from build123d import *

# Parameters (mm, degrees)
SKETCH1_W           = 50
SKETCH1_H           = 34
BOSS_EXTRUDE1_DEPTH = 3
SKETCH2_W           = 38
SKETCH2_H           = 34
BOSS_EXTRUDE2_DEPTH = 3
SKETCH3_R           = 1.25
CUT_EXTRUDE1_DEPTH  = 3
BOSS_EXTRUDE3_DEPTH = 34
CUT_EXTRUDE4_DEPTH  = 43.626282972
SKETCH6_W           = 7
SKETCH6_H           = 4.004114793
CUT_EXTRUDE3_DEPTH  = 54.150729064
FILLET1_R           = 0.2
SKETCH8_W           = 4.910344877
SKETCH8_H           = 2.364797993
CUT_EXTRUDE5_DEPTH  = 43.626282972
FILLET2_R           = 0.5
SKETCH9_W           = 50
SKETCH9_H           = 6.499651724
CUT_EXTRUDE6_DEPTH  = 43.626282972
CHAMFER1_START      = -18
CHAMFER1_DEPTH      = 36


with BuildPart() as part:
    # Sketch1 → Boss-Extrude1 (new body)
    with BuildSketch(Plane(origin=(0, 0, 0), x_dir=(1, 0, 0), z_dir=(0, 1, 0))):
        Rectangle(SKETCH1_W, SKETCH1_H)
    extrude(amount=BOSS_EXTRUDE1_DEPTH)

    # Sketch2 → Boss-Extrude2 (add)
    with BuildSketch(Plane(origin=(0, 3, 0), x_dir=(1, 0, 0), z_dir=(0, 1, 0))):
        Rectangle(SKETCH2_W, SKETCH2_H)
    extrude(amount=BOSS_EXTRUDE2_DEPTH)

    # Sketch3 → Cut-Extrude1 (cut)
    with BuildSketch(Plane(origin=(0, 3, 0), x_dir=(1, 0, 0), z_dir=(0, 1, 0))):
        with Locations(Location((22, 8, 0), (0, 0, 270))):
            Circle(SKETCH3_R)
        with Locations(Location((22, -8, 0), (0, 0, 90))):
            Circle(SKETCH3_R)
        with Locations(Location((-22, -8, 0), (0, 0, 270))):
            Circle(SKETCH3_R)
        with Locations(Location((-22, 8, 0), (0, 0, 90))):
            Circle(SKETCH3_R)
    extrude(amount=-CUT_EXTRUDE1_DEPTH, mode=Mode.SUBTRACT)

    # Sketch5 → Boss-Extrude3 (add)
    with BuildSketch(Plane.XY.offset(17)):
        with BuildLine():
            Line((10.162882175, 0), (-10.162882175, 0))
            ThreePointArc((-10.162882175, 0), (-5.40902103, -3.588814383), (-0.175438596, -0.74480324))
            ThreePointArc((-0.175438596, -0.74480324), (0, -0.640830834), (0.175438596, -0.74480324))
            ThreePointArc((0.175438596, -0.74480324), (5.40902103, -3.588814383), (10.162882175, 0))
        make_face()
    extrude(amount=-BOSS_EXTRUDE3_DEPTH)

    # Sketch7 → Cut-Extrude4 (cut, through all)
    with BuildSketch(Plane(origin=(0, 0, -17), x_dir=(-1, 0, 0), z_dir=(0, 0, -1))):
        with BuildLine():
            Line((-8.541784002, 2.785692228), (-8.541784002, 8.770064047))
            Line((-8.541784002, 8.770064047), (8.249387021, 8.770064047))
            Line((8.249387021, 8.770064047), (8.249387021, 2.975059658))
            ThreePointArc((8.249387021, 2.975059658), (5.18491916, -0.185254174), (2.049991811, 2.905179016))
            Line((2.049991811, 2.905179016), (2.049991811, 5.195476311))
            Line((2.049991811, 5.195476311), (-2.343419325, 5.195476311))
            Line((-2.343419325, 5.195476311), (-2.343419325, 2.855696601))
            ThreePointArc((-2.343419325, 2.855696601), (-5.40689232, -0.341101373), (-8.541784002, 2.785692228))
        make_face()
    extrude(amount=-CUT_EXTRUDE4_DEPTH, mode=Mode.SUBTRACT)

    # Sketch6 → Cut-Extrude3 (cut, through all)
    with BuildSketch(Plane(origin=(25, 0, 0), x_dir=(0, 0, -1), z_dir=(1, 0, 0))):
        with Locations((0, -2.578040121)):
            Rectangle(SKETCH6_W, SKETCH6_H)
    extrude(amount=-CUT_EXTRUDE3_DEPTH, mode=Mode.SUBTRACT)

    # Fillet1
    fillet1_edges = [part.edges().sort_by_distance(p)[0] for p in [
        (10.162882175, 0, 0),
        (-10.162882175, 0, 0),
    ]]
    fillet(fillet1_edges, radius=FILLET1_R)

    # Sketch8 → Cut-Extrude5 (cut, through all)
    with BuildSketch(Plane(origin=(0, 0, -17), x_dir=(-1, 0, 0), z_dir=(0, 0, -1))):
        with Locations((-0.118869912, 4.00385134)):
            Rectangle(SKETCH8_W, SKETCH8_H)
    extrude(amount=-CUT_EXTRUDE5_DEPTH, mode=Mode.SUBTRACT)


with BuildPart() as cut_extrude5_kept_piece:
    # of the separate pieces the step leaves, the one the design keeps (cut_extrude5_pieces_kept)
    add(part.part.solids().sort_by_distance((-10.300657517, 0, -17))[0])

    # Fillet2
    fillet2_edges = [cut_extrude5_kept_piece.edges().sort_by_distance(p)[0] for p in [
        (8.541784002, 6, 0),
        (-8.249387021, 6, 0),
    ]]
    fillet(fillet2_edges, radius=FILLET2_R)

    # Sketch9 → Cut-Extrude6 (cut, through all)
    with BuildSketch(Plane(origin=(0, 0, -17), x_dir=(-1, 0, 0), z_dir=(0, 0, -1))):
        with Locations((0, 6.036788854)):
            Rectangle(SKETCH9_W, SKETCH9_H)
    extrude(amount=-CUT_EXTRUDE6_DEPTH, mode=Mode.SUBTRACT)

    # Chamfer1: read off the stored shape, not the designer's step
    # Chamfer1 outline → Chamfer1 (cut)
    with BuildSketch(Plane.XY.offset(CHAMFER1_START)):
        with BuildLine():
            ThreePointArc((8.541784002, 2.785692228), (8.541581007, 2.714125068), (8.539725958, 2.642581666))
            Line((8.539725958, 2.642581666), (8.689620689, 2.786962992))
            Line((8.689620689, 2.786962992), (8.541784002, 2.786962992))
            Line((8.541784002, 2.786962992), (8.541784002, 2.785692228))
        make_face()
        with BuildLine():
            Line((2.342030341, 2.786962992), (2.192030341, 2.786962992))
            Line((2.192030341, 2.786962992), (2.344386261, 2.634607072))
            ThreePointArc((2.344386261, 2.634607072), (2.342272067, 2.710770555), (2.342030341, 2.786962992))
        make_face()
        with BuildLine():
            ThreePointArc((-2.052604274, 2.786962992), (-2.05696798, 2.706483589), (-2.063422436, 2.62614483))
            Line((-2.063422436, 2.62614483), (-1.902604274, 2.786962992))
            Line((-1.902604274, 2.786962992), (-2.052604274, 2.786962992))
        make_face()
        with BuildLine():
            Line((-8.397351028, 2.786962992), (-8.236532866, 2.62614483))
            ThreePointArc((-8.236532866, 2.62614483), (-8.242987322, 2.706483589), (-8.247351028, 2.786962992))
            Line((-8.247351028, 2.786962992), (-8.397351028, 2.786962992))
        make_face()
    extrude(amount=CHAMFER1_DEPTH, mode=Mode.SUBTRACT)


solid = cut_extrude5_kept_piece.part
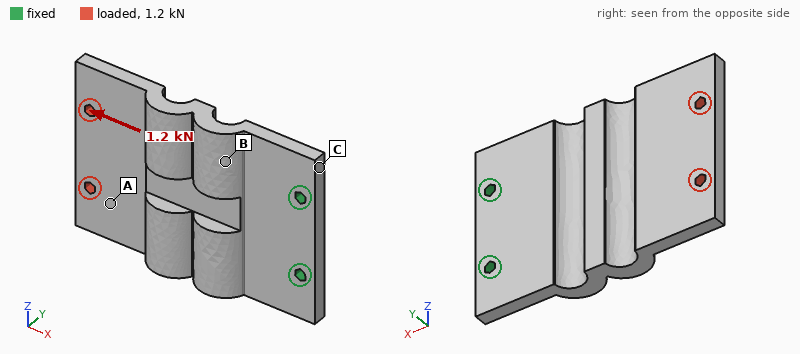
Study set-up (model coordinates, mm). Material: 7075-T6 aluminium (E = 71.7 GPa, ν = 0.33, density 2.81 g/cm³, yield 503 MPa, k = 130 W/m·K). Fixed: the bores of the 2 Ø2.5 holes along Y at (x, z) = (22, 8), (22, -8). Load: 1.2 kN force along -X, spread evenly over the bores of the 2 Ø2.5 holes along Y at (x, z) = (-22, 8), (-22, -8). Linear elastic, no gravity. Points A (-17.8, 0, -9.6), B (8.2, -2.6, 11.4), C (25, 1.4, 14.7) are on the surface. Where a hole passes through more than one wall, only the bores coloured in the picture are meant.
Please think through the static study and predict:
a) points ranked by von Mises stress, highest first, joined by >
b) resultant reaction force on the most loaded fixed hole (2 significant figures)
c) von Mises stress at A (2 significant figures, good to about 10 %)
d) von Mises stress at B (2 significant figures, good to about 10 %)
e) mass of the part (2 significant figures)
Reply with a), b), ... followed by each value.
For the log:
a) B > A > C
b) 600 N
c) 22 MPa
d) 46 MPa
e) 15 g
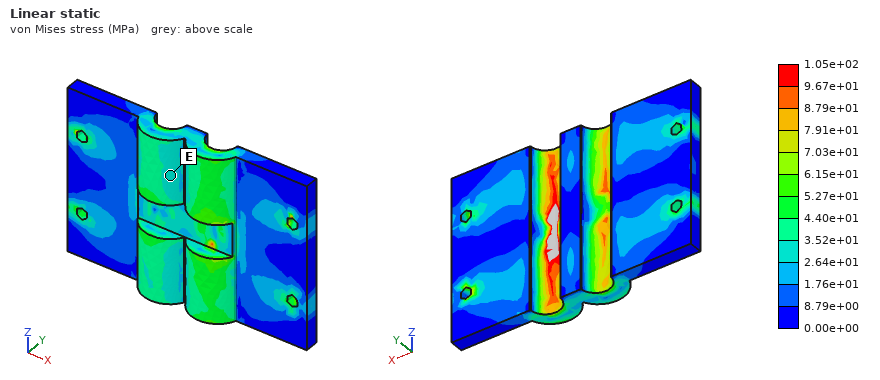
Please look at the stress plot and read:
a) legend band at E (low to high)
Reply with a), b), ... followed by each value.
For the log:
a) 2.64e+01 to 3.52e+01 MPa
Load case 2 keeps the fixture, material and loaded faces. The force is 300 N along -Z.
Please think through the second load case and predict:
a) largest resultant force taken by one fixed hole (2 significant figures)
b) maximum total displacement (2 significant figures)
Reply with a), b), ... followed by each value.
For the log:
a) 750 N
b) 79 µm
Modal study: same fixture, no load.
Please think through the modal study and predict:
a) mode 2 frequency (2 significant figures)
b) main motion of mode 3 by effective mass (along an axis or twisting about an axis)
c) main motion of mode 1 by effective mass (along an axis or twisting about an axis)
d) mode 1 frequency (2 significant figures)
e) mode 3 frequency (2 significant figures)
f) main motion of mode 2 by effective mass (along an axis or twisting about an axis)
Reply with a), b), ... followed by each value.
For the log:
a) 3000 Hz
b) along Y
c) along Y
d) 950 Hz
e) 5600 Hz
f) twisting about X
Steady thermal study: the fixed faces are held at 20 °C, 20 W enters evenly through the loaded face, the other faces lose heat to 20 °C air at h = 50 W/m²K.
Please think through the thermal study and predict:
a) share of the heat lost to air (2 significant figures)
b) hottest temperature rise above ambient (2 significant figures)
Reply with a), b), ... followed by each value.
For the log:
a) 33 %
b) 69 K
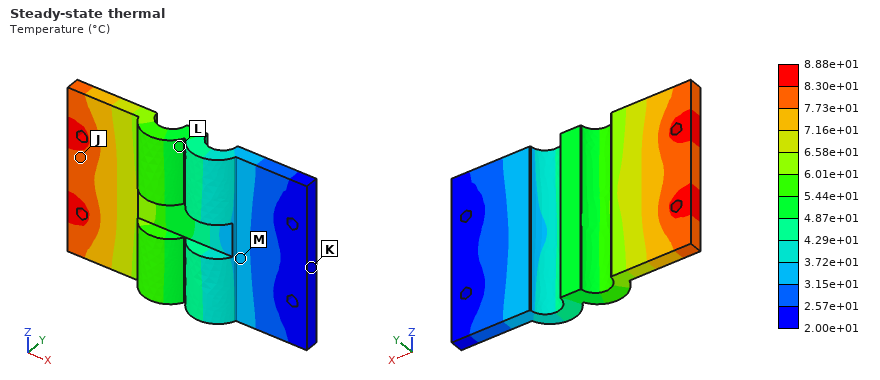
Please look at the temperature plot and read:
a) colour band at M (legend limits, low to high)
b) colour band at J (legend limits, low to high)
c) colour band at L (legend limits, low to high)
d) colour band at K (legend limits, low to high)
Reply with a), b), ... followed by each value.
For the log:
a) 3.15e+01 to 3.72e+01 °C
b) 7.73e+01 to 8.30e+01 °C
c) 4.87e+01 to 5.44e+01 °C
d) 2.00e+01 to 2.57e+01 °C
